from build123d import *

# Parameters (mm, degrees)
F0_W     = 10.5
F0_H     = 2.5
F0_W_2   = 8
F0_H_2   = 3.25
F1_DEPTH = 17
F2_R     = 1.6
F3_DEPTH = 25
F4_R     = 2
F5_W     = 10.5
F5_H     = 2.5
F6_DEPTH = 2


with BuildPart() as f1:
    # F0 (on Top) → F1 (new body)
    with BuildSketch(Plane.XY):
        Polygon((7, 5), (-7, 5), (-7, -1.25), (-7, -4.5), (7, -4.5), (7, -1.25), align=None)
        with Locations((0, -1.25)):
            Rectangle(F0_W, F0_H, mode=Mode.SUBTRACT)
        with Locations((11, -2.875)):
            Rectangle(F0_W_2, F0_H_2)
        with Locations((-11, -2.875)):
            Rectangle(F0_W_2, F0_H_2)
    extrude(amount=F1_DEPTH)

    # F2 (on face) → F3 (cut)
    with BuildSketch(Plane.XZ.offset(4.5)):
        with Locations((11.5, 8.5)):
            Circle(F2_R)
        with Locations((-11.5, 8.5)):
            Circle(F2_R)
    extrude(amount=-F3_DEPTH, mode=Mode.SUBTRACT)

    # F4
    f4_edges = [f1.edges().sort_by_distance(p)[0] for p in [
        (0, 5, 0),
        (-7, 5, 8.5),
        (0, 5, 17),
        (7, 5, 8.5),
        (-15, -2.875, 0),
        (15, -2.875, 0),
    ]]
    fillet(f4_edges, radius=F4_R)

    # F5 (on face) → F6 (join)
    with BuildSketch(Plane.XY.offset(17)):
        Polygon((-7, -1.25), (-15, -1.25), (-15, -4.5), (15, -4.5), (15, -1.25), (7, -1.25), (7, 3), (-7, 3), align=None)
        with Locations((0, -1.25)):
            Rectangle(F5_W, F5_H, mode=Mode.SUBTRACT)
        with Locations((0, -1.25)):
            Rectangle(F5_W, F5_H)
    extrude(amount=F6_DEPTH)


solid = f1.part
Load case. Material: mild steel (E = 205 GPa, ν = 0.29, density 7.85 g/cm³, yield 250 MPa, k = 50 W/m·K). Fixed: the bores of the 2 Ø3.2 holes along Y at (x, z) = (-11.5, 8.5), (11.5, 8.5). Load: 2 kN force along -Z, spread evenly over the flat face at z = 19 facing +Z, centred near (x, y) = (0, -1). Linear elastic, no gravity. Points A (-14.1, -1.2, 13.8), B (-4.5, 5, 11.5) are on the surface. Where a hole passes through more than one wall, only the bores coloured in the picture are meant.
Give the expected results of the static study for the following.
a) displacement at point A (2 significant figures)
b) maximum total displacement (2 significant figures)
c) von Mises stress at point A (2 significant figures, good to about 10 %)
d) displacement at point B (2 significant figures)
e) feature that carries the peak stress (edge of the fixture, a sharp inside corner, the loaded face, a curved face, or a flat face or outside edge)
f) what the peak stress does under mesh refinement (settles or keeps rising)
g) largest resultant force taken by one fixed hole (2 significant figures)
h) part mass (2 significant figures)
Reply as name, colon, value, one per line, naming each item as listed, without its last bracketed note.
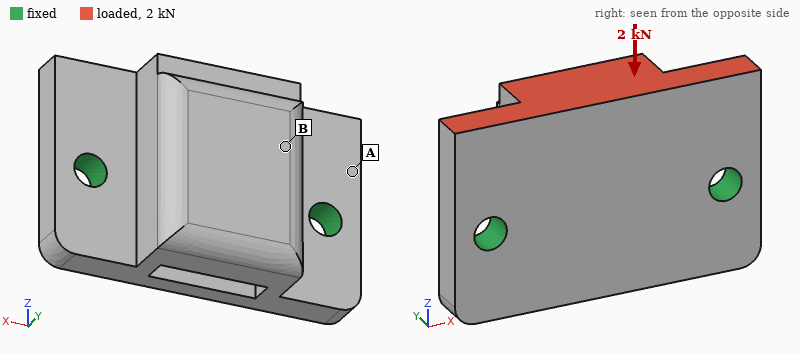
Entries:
displacement at point A: 1.2 µm
maximum total displacement: 7.2 µm
von Mises stress at point A: 29 MPa
displacement at point B: 5.8 µm
feature that carries the peak stress: edge of the fixture
what the peak stress does under mesh refinement: keeps rising
largest resultant force taken by one fixed hole: 1.0 kN
part mass: 23 g
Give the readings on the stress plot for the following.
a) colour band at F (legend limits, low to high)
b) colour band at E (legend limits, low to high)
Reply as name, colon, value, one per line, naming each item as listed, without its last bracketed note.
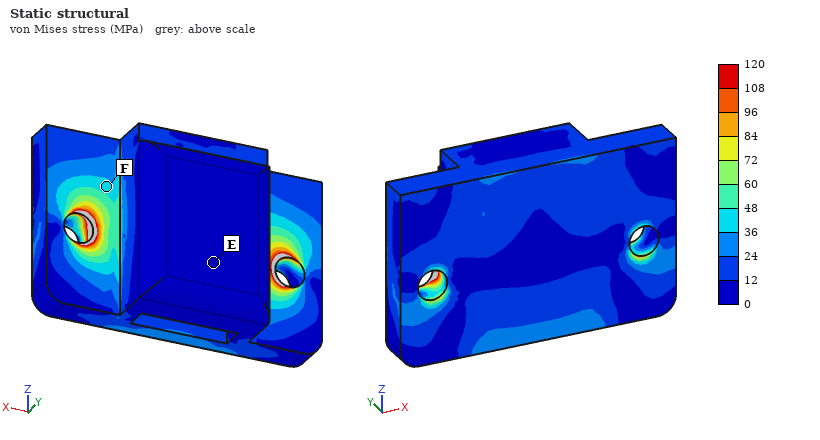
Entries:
colour band at F: 36 to 48 MPa
colour band at E: 0 to 12 MPa
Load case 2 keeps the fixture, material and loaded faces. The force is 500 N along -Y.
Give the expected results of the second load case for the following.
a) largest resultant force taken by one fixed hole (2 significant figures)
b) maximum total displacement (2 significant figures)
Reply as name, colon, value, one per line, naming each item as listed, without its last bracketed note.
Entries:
largest resultant force taken by one fixed hole: 260 N
maximum total displacement: 11 µm
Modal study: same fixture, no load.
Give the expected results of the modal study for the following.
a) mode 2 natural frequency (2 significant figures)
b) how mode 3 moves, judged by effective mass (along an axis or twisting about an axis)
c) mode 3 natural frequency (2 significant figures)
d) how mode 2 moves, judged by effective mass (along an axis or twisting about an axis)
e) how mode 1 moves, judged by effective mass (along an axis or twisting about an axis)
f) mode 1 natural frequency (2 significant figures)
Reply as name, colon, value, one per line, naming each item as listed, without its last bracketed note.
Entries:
mode 2 natural frequency: 24 kHz
how mode 3 moves, judged by effective mass: along X
mode 3 natural frequency: 32 kHz
how mode 2 moves, judged by effective mass: along Y
how mode 1 moves, judged by effective mass: along Z
mode 1 natural frequency: 13 kHz
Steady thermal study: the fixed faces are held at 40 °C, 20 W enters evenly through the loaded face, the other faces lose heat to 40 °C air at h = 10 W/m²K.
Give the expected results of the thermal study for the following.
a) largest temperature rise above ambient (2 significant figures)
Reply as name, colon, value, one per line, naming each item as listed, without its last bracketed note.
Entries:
largest temperature rise above ambient: 47 K
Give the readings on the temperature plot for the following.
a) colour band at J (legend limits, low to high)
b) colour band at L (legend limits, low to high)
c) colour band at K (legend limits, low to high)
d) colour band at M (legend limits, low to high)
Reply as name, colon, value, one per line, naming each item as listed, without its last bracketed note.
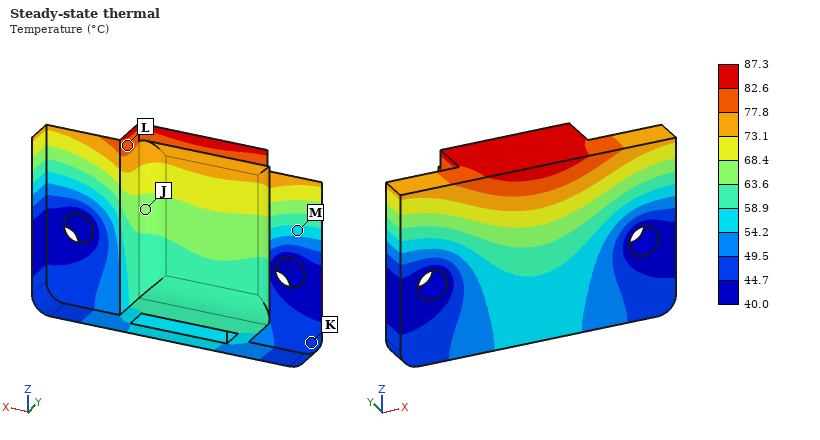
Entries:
colour band at J: 63.6 to 68.4 °C
colour band at L: 77.8 to 82.6 °C
colour band at K: 44.7 to 49.5 °C
colour band at M: 54.2 to 58.9 °C
